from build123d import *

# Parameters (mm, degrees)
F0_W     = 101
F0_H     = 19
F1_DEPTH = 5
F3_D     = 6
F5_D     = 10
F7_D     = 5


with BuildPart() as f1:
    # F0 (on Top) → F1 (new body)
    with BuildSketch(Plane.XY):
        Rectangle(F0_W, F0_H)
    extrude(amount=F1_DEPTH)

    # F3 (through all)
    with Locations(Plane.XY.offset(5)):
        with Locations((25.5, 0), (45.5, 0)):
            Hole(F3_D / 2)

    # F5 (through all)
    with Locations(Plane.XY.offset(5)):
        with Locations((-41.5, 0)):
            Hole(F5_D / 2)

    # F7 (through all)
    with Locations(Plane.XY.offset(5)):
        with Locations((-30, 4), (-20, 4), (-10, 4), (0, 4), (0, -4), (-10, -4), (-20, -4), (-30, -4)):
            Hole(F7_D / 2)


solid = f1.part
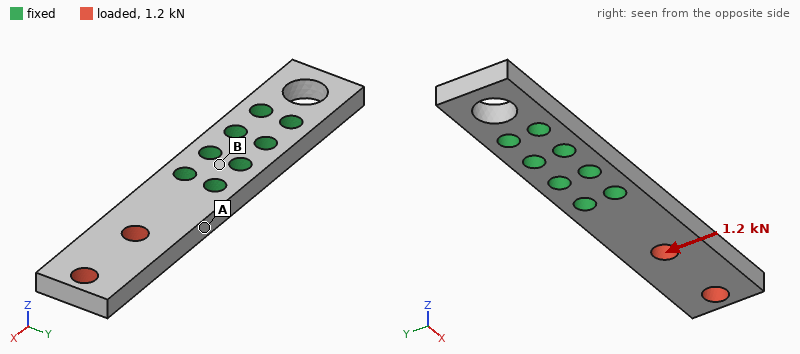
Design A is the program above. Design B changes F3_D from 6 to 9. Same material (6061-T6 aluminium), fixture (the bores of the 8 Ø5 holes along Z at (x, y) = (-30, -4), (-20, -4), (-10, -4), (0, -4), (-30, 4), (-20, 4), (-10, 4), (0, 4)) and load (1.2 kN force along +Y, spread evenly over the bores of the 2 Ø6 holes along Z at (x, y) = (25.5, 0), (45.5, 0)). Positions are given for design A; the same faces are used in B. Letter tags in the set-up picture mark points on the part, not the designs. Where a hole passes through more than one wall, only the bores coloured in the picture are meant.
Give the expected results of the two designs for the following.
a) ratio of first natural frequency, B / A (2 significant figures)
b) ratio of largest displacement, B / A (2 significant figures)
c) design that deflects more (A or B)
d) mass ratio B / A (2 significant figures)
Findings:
1.1
1.1
B
0.96
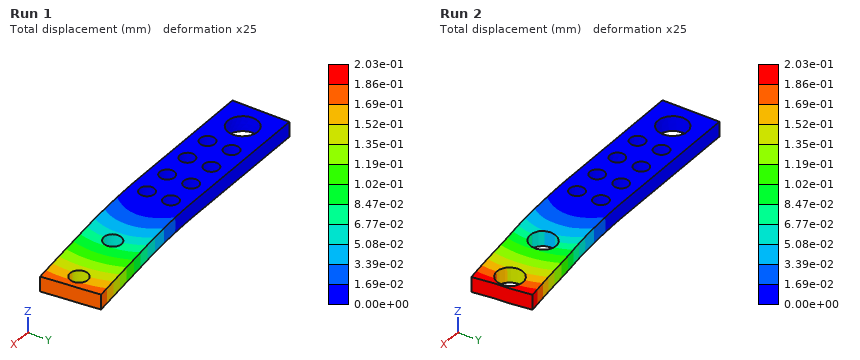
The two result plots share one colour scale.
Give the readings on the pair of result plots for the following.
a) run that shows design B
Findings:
Run 2
